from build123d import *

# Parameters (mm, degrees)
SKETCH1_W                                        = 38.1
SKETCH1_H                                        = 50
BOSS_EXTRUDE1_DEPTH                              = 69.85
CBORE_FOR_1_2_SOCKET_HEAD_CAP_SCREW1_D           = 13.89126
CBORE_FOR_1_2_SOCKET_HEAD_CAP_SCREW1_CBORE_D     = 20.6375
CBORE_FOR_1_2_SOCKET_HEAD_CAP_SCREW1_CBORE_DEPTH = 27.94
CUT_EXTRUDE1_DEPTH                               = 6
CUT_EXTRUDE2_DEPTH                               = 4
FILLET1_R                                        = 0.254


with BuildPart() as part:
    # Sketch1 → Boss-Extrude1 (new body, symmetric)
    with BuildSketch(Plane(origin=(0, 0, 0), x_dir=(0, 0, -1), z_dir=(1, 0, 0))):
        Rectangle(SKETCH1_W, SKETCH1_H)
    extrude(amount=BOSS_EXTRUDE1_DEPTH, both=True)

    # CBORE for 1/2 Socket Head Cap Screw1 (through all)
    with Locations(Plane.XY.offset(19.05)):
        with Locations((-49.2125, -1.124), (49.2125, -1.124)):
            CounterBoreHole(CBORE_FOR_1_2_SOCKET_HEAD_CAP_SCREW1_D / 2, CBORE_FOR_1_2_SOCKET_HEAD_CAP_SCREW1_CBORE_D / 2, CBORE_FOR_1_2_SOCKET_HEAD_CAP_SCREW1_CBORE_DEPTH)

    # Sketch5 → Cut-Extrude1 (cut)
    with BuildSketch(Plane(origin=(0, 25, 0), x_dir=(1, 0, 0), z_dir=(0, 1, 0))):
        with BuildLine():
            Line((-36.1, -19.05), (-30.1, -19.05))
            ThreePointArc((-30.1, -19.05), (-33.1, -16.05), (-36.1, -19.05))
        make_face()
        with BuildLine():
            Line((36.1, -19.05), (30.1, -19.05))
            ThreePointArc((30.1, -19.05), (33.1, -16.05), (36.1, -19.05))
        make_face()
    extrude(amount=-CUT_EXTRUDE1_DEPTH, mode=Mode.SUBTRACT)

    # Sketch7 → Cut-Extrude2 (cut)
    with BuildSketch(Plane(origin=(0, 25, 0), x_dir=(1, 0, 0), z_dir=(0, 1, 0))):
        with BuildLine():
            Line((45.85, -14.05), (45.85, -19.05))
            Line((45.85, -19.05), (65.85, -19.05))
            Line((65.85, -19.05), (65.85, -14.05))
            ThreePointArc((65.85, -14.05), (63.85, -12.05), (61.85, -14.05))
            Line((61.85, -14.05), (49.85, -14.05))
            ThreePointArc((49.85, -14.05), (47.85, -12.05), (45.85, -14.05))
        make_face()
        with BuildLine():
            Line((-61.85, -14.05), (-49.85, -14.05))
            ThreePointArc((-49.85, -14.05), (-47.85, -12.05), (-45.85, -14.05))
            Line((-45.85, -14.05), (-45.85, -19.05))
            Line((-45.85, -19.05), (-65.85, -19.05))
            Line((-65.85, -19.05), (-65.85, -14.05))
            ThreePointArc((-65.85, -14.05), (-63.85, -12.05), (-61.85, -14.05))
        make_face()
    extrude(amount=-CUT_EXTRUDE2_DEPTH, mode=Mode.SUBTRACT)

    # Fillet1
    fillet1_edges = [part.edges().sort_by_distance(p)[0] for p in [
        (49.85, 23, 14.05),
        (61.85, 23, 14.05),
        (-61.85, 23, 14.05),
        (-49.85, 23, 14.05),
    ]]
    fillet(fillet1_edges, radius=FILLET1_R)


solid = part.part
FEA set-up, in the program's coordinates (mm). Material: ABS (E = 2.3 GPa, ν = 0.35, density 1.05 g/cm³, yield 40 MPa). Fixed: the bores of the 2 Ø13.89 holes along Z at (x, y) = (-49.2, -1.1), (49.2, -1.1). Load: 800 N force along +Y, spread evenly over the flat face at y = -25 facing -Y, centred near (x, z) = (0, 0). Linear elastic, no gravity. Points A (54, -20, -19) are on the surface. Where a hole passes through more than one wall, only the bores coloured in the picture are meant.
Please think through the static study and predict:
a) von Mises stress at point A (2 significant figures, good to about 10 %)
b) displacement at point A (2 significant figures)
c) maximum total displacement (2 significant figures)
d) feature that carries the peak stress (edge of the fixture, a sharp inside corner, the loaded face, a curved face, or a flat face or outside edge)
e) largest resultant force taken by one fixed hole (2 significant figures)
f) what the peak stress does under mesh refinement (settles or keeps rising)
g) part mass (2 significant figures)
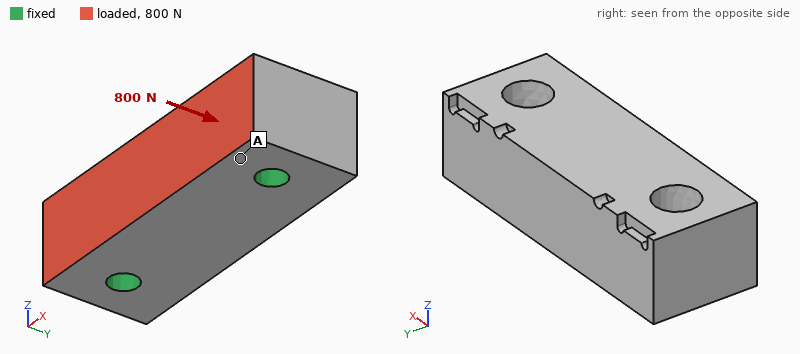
0.53 MPa
27 µm
78 µm
edge of the fixture
400 N
keeps rising
260 g
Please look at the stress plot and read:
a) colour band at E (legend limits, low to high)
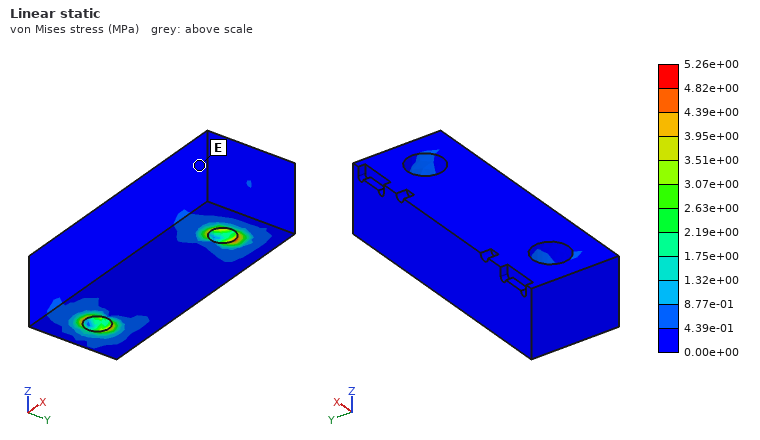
0.00e+00 to 4.39e-01 MPa
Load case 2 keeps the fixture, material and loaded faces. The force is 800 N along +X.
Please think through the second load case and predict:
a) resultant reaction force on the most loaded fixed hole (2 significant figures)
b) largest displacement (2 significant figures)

450 N
25 µm
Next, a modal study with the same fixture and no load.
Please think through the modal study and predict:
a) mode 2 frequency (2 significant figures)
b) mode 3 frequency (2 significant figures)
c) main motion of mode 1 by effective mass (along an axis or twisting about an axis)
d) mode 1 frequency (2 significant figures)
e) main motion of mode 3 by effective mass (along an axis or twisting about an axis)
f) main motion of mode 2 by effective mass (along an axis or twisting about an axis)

2300 Hz
2600 Hz
along Y
1100 Hz
twisting about Z
along Z
